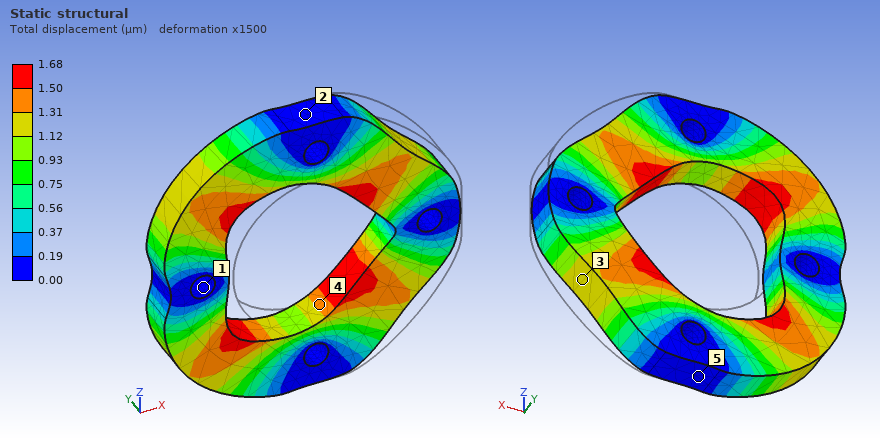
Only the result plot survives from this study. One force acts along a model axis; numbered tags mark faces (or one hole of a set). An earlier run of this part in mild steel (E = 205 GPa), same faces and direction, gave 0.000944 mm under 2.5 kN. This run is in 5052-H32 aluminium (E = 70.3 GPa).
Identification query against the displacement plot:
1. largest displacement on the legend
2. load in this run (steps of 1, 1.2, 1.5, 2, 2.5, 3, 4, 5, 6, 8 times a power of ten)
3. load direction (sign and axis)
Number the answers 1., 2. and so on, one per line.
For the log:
1. 1.68 µm
2. 1.5 kN
3. -X
